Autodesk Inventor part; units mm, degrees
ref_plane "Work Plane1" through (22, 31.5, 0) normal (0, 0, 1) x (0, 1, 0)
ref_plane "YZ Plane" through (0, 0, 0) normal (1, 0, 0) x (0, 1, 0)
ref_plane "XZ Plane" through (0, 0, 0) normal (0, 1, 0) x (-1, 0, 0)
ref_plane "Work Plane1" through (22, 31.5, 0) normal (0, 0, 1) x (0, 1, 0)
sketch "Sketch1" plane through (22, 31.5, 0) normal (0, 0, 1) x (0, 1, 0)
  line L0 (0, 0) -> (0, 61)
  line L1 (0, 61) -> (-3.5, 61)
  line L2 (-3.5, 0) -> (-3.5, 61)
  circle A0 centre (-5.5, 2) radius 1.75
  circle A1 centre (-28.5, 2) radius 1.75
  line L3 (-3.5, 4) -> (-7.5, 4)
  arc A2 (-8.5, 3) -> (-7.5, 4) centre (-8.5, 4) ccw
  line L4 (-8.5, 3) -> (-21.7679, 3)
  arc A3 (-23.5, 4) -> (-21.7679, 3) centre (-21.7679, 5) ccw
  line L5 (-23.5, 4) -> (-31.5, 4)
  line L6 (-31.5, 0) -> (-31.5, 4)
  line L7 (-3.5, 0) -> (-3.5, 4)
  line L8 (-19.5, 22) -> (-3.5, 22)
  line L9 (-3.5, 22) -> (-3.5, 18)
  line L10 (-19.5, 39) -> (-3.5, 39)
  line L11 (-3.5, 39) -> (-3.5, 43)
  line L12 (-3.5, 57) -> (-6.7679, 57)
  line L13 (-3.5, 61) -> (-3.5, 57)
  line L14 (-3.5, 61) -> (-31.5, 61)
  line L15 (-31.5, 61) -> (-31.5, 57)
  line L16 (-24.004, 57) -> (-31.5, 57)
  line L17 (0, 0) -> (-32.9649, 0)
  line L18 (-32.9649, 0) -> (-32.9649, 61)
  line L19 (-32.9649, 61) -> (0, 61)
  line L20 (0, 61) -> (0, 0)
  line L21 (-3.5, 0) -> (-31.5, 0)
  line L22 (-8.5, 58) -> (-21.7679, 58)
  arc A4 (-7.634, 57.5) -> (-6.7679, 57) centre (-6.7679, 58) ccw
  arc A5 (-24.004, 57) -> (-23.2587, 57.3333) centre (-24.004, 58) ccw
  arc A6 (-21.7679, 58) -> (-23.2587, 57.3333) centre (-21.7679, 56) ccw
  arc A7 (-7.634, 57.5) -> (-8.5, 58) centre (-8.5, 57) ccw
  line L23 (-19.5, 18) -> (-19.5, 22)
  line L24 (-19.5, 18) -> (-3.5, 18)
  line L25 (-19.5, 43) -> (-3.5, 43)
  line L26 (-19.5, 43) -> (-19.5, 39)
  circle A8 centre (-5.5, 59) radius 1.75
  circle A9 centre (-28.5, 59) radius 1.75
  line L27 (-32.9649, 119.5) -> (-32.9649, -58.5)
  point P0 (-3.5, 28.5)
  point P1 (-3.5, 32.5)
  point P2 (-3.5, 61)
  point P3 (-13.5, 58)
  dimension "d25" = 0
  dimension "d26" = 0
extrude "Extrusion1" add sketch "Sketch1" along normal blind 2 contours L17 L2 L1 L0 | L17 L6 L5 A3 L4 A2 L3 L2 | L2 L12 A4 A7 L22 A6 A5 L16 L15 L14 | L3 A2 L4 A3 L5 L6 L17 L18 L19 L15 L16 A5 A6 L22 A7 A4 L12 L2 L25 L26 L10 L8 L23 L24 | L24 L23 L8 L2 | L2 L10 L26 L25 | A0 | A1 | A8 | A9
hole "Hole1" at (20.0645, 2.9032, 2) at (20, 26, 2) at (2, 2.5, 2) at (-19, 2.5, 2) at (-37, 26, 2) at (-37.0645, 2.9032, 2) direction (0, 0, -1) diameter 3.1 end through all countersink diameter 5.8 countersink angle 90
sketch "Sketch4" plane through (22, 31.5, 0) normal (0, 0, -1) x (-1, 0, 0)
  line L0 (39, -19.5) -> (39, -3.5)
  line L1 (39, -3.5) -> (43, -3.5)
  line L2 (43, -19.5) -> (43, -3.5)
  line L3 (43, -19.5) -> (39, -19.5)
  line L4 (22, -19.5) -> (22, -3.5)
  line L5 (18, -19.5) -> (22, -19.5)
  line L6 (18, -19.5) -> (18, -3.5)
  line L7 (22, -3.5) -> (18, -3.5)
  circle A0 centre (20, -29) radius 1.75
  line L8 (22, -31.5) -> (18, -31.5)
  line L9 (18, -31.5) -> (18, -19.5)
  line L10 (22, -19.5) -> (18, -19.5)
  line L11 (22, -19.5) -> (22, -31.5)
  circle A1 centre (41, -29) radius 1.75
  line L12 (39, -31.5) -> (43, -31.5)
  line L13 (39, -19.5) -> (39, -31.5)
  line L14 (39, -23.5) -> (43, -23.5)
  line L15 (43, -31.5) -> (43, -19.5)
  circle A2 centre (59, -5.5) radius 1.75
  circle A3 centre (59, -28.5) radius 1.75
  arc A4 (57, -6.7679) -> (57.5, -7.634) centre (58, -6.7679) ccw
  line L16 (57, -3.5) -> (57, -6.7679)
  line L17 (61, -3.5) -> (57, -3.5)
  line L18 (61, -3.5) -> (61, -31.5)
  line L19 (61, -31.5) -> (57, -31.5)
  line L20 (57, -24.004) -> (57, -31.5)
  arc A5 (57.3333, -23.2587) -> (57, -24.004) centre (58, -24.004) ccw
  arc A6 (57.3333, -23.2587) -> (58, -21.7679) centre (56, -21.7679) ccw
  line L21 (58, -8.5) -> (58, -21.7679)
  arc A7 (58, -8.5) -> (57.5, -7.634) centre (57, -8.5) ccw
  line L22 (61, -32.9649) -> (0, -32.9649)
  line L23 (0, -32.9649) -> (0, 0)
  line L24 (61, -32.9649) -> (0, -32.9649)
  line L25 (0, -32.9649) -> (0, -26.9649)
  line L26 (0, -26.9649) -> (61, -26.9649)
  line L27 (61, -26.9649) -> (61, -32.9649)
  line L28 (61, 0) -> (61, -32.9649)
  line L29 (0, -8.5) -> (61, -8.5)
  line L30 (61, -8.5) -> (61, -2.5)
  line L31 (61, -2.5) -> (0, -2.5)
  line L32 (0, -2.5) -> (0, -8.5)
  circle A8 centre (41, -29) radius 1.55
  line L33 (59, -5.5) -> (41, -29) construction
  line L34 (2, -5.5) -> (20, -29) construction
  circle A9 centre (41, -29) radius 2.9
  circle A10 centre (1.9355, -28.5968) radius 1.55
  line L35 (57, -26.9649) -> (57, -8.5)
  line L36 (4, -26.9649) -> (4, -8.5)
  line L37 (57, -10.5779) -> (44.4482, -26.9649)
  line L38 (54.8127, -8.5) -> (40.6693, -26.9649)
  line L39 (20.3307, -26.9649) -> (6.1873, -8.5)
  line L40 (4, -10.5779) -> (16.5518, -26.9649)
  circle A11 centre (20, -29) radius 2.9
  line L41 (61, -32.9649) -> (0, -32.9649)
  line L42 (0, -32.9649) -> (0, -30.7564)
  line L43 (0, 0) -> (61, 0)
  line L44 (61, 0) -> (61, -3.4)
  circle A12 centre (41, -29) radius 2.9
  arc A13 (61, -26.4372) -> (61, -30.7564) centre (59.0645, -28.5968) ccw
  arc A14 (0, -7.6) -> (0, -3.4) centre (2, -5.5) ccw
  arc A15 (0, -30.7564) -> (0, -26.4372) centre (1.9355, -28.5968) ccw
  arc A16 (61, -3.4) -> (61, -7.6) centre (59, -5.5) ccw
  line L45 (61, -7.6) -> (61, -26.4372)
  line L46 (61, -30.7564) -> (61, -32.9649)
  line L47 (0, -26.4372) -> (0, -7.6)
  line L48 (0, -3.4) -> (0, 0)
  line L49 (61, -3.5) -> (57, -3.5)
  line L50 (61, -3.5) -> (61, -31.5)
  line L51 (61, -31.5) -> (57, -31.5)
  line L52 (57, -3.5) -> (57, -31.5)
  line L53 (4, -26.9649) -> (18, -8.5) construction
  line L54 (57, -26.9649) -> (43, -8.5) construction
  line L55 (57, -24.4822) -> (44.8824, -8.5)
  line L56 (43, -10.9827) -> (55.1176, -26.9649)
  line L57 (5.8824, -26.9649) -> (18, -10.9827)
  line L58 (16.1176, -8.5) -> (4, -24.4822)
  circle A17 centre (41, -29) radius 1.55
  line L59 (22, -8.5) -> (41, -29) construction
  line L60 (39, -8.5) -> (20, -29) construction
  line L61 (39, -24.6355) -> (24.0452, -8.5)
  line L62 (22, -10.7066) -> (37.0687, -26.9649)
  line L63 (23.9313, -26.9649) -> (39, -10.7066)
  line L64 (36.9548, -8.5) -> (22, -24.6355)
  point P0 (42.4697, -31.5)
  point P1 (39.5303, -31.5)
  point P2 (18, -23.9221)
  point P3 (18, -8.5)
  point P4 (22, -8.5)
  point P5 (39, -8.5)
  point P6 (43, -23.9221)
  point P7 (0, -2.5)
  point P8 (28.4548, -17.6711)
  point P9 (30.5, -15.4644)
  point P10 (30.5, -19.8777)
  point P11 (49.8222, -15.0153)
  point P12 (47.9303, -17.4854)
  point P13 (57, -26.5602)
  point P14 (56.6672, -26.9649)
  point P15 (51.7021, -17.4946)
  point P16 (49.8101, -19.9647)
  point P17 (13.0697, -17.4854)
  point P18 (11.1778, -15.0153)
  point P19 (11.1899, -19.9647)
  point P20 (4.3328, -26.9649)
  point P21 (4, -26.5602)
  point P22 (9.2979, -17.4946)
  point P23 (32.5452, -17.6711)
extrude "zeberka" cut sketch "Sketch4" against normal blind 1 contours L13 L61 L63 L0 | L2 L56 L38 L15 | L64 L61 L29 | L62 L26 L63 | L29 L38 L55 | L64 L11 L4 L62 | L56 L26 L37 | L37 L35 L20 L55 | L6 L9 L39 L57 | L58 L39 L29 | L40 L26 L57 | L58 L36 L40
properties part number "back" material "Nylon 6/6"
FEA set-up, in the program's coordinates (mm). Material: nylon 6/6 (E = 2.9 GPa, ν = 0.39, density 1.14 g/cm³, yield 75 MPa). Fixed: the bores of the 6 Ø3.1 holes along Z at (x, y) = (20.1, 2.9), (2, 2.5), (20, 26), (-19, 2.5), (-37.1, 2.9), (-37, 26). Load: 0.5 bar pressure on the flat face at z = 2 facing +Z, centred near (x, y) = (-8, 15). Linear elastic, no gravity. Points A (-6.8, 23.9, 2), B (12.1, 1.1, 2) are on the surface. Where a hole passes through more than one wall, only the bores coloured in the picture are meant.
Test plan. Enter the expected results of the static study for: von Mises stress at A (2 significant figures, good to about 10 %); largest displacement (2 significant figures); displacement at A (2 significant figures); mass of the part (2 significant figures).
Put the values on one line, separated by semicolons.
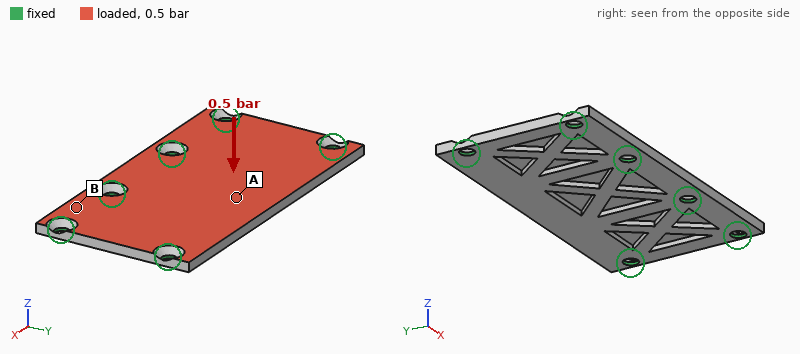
7.7 MPa; 0.82 mm; 0.61 mm; 3.9 g
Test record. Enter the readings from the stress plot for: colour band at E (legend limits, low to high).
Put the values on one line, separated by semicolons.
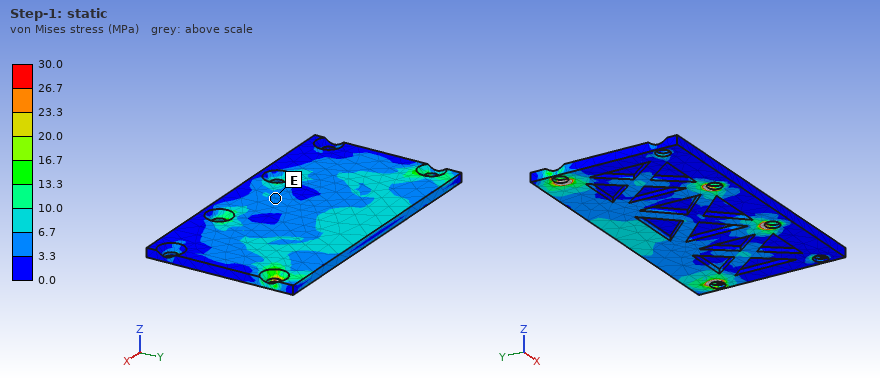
3.3 to 6.7 MPa
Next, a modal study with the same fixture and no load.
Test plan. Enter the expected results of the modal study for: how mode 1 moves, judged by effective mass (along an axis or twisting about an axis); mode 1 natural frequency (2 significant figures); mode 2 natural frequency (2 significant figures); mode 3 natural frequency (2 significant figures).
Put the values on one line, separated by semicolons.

along Z; 1100 Hz; 2600 Hz; 3400 Hz
